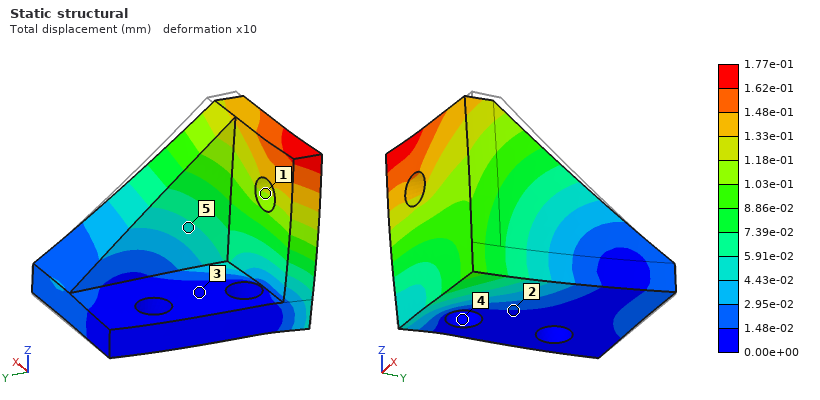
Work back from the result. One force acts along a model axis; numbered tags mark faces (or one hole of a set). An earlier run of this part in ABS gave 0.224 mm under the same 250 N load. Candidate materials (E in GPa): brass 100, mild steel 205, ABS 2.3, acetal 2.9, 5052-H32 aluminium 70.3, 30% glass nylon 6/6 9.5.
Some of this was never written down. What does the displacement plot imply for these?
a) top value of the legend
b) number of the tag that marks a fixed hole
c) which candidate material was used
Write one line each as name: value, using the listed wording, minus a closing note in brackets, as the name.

top value of the legend: 1.77e-01 mm
number of the tag that marks a fixed hole: 4
which candidate material was used: acetal
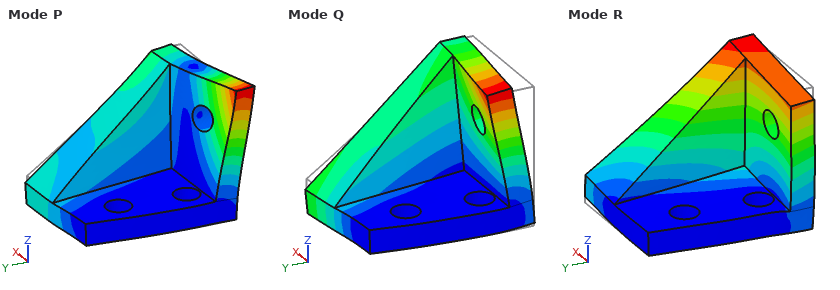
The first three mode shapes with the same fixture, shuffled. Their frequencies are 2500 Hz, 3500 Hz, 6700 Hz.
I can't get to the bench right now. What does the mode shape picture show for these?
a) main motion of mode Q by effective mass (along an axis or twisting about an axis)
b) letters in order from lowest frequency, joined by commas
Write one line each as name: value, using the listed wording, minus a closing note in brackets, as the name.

main motion of mode Q by effective mass: along Y
letters in order from lowest frequency, joined by commas: R, Q, P
